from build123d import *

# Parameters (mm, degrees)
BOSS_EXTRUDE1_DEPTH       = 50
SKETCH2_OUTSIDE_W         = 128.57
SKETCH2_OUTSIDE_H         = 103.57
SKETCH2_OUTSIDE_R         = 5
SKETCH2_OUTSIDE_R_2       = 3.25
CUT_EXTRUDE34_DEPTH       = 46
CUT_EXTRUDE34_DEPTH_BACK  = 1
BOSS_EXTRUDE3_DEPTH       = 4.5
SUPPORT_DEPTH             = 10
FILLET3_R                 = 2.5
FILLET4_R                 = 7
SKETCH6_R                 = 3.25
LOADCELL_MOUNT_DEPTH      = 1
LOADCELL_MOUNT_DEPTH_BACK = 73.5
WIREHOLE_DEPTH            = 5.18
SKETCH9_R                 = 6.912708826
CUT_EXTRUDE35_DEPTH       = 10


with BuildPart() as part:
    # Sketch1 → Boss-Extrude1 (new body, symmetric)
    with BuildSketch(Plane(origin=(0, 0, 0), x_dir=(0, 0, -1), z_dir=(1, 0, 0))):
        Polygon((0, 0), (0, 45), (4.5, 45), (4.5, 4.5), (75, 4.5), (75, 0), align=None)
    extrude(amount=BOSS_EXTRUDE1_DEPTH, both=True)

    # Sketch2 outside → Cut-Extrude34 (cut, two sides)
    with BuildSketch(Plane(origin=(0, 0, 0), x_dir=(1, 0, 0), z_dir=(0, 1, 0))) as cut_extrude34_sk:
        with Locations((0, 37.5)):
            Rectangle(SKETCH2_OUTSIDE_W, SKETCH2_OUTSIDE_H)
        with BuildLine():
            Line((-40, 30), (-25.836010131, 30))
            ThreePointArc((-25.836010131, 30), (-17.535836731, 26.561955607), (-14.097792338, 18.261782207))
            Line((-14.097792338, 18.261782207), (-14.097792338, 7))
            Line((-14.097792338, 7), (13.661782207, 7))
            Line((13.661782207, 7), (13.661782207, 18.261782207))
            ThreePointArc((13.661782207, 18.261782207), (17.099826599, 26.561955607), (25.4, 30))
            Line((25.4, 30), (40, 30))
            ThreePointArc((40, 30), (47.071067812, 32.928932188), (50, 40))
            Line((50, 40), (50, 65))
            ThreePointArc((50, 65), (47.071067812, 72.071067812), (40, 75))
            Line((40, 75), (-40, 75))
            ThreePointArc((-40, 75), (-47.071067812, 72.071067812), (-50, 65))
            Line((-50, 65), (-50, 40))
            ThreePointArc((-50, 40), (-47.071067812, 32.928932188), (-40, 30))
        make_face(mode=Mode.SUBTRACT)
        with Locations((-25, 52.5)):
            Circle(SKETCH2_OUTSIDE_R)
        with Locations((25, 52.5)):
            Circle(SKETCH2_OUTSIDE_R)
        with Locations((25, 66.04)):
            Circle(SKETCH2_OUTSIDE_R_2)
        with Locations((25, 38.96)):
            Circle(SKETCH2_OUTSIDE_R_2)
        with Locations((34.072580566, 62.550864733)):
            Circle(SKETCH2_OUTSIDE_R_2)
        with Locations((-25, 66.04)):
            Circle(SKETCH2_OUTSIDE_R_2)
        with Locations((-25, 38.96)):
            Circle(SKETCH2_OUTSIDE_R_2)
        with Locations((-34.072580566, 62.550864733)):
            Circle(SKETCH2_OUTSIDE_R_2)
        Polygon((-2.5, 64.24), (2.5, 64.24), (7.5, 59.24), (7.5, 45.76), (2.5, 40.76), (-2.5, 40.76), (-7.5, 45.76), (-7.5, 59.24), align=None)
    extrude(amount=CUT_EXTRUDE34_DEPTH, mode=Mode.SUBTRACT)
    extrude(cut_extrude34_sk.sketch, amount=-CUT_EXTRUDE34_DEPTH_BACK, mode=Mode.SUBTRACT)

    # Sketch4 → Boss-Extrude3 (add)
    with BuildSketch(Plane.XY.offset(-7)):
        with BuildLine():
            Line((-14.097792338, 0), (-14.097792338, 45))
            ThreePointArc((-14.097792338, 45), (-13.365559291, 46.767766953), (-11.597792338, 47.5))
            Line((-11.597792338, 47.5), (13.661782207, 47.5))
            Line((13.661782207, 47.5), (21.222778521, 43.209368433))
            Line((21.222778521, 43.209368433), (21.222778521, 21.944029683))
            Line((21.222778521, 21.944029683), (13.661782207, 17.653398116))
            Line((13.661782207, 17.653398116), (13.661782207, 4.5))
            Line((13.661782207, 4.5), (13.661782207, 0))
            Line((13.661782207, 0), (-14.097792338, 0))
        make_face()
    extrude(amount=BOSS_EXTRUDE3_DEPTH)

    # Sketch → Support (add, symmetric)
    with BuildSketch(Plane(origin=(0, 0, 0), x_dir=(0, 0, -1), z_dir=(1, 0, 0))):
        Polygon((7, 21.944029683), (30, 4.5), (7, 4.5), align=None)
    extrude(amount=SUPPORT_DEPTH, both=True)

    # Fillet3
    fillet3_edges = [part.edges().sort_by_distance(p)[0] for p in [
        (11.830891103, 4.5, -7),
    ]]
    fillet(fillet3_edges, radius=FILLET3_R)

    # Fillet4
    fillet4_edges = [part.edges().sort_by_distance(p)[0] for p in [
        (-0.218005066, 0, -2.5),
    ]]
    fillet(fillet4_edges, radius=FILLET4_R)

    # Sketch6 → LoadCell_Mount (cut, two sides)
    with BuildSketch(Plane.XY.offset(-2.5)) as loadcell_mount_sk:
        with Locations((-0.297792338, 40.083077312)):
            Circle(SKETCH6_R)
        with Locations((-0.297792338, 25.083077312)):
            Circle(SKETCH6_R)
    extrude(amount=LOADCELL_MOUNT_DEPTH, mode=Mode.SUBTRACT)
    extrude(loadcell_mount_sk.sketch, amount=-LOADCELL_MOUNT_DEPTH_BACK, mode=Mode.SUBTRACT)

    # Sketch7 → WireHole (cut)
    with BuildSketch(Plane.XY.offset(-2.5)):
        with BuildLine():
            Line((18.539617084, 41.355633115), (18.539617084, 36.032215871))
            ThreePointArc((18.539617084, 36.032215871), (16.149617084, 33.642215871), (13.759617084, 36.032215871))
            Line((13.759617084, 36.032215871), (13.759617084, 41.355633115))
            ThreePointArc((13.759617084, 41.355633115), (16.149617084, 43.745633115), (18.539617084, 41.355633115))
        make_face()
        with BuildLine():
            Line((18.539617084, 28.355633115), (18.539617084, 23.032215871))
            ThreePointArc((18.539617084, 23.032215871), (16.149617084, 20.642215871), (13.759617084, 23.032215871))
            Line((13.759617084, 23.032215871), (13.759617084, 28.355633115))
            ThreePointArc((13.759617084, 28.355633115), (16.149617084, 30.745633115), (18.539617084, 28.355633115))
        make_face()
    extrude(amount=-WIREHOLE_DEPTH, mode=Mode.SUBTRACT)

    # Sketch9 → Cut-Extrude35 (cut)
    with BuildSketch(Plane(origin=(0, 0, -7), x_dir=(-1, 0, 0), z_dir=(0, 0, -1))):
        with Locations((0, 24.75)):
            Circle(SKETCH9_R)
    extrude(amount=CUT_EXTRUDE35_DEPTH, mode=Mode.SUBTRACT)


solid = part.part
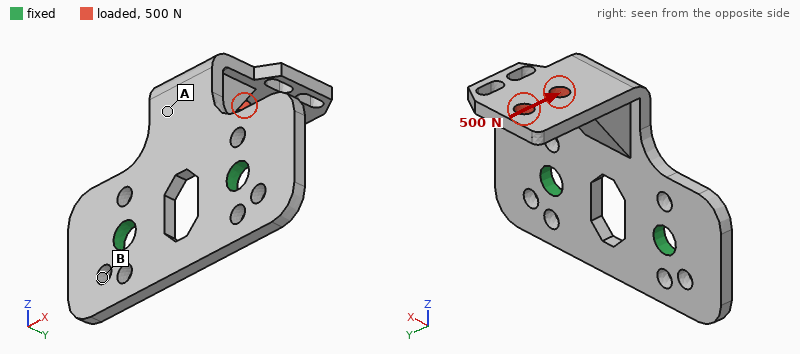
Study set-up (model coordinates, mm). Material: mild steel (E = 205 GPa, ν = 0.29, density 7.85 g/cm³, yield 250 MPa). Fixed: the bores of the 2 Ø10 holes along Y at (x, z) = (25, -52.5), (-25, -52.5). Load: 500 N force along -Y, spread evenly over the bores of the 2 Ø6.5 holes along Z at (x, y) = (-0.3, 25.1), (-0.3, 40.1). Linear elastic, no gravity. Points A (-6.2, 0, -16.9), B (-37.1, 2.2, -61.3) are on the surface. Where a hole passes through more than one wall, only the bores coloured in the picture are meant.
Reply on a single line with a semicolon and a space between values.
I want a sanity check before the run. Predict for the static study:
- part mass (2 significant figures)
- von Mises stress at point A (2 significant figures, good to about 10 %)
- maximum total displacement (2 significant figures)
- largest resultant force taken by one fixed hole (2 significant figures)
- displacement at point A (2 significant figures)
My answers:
230 g; 23 MPa; 0.34 mm; 250 N; 0.13 mm
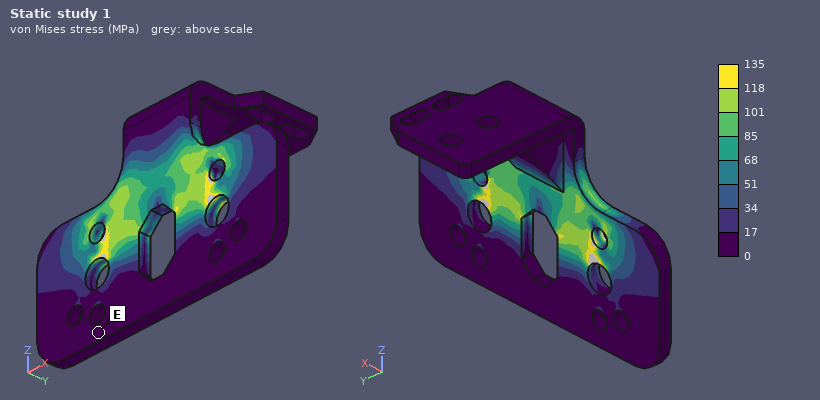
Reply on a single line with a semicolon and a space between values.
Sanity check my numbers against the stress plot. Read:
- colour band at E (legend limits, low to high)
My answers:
0 to 17 MPa
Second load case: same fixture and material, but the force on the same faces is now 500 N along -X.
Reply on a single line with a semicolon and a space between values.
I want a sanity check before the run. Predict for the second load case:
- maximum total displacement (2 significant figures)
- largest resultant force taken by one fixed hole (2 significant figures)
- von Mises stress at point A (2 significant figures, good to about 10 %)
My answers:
93 µm; 650 N; 22 MPa
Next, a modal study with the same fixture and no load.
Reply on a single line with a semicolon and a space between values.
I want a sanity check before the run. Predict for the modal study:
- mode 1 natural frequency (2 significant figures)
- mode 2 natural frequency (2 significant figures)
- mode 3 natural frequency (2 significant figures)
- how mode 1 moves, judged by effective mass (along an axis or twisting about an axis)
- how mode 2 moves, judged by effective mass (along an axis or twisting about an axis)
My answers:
780 Hz; 2200 Hz; 3300 Hz; along Y; along X
